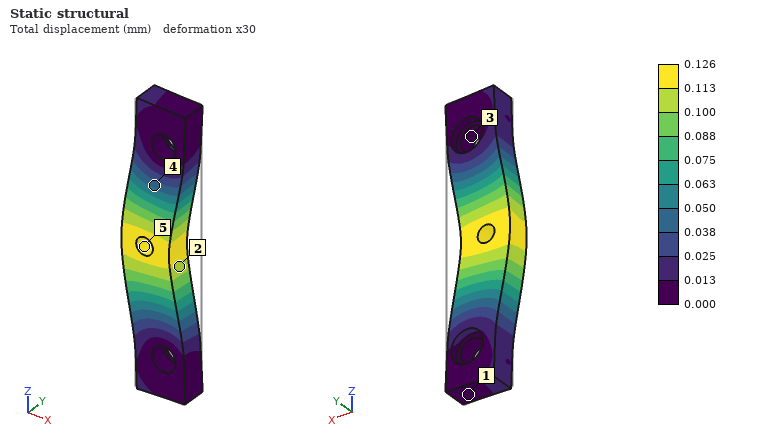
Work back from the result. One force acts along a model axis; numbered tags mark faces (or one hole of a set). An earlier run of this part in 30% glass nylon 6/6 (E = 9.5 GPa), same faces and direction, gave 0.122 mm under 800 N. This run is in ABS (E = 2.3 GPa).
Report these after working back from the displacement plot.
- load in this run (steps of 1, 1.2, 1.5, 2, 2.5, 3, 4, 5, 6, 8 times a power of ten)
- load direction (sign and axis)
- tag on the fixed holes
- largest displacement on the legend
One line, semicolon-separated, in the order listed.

200 N; -X; 3; 0.126 mm
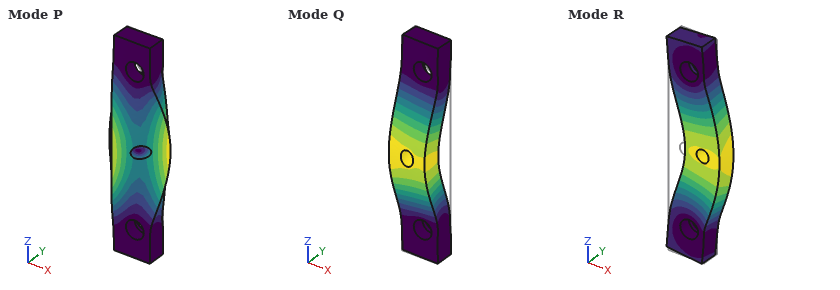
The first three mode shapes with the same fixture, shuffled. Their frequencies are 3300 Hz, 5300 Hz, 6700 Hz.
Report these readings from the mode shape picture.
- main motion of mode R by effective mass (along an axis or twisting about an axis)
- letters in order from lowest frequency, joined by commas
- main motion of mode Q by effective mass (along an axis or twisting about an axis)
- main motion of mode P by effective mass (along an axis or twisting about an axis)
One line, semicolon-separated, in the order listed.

along X; Q, R, P; along Y; twisting about Z
